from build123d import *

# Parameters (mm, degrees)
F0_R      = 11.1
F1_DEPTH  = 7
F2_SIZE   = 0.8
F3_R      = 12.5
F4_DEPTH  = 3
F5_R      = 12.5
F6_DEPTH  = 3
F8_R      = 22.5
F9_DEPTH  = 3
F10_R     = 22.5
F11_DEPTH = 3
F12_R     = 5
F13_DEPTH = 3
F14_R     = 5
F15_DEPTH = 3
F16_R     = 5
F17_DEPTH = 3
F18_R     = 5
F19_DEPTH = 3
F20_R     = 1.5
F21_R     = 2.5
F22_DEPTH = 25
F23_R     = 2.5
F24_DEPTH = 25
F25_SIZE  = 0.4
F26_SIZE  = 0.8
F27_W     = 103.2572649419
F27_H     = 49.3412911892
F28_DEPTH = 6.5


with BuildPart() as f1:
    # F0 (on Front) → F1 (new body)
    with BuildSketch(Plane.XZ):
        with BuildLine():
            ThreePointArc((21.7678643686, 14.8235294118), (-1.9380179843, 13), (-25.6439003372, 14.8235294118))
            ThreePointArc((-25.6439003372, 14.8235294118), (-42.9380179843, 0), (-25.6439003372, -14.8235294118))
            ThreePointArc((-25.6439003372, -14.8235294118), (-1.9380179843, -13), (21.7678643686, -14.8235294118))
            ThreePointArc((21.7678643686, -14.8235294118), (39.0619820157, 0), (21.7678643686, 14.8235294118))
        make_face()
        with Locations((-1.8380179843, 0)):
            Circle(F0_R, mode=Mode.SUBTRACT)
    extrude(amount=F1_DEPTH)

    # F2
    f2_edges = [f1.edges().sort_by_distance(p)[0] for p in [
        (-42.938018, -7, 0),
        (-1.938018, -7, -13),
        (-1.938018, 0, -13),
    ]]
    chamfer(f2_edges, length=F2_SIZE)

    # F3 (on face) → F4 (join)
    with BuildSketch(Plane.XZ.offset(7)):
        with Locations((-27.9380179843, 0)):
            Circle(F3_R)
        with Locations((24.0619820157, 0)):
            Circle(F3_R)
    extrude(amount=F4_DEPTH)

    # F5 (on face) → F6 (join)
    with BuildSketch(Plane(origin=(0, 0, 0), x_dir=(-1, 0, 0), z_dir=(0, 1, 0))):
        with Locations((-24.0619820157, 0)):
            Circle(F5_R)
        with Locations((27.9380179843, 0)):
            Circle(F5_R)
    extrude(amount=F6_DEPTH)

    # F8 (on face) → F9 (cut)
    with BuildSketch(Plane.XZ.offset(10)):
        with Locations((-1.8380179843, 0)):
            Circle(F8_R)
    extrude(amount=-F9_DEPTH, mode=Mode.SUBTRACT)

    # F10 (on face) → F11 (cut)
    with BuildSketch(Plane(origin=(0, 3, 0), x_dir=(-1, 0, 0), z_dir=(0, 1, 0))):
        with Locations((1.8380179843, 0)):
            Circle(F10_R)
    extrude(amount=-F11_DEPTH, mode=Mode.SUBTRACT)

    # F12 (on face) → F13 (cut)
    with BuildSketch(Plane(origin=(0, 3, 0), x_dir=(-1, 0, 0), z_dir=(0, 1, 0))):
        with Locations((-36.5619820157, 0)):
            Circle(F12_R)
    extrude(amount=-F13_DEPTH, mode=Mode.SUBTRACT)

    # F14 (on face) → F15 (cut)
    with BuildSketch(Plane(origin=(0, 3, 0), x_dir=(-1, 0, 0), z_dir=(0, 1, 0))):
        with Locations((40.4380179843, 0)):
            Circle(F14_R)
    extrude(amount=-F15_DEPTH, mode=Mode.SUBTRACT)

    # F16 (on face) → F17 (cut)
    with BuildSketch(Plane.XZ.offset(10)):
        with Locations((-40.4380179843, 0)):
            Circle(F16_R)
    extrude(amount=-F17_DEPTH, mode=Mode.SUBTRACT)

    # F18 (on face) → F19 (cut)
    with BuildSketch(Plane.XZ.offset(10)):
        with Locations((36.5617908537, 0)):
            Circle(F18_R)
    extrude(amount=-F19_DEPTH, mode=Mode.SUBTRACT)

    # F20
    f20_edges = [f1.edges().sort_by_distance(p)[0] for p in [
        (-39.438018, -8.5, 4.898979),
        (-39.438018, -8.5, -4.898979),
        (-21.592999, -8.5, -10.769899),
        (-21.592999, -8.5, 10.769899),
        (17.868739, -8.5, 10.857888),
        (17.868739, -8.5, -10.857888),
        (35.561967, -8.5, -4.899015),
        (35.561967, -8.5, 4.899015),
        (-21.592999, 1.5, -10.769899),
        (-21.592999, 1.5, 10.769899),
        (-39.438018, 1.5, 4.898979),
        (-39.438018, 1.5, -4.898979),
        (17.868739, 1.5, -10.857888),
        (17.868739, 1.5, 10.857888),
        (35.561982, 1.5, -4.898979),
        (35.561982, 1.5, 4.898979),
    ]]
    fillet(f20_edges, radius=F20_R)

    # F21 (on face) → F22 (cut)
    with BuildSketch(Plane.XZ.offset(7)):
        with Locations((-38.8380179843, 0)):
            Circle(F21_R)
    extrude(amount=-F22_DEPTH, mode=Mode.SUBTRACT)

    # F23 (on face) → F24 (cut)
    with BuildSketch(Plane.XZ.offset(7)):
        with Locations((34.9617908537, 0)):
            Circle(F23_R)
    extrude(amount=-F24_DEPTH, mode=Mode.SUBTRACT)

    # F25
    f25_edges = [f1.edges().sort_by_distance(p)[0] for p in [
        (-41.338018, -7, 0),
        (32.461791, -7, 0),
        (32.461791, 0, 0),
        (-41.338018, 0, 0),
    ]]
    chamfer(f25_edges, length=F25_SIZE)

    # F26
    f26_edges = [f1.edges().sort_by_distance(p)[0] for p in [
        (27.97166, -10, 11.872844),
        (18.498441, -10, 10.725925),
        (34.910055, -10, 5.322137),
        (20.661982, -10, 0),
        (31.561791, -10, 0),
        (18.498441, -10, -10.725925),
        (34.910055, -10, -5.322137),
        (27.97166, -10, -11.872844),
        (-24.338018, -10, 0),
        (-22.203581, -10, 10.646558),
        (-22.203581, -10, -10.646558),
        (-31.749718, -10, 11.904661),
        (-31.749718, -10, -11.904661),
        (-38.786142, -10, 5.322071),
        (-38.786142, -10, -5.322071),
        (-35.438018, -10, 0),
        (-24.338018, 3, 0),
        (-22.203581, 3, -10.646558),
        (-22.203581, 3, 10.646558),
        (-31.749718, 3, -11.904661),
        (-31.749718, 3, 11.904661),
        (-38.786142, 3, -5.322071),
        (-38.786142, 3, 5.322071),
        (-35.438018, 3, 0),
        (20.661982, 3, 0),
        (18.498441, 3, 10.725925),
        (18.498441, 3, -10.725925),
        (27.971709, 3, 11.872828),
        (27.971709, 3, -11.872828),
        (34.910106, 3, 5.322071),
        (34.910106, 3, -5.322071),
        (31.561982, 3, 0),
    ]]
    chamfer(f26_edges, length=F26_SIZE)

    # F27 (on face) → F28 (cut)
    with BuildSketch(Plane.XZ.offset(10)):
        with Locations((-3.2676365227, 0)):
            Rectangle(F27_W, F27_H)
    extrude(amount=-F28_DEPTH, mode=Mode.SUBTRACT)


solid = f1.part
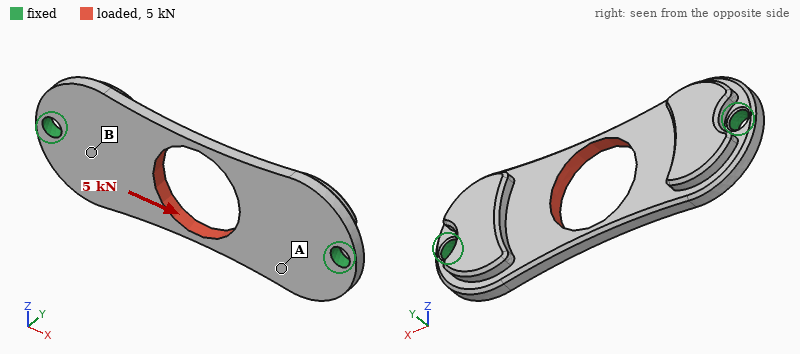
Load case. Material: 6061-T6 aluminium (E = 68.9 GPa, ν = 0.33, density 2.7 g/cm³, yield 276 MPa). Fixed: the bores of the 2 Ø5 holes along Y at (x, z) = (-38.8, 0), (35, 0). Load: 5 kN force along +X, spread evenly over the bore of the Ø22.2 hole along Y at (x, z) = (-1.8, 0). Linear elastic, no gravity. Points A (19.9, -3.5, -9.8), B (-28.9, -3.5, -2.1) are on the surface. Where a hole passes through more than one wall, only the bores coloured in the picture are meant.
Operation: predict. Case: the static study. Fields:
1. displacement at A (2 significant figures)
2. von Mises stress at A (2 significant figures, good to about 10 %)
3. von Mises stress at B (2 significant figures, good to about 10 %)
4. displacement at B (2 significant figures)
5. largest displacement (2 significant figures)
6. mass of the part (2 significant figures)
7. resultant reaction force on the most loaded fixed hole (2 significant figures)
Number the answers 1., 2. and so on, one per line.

1. 10 µm
2. 25 MPa
3. 45 MPa
4. 6.4 µm
5. 20 µm
6. 21 g
7. 2.5 kN
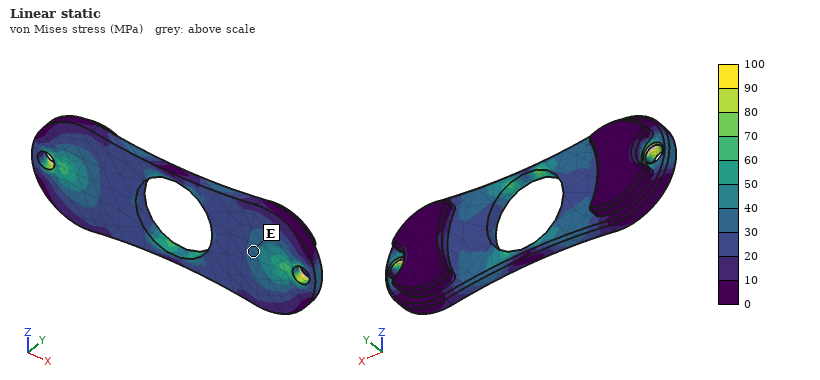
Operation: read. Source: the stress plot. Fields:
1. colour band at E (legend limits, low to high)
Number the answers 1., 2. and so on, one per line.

1. 30 to 40 MPa
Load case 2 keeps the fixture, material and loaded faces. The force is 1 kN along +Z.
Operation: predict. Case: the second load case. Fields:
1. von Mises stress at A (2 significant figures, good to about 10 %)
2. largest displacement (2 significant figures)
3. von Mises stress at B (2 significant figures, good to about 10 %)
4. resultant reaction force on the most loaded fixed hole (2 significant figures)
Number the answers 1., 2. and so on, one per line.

1. 9.3 MPa
2. 31 µm
3. 16 MPa
4. 500 N
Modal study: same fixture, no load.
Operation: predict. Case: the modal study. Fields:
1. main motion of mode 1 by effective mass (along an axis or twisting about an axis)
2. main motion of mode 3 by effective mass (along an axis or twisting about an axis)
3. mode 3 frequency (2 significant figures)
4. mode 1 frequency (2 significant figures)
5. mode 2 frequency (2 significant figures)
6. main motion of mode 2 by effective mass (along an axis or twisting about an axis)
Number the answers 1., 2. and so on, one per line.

1. along Y
2. twisting about Z
3. 7500 Hz
4. 4200 Hz
5. 7000 Hz
6. twisting about X
